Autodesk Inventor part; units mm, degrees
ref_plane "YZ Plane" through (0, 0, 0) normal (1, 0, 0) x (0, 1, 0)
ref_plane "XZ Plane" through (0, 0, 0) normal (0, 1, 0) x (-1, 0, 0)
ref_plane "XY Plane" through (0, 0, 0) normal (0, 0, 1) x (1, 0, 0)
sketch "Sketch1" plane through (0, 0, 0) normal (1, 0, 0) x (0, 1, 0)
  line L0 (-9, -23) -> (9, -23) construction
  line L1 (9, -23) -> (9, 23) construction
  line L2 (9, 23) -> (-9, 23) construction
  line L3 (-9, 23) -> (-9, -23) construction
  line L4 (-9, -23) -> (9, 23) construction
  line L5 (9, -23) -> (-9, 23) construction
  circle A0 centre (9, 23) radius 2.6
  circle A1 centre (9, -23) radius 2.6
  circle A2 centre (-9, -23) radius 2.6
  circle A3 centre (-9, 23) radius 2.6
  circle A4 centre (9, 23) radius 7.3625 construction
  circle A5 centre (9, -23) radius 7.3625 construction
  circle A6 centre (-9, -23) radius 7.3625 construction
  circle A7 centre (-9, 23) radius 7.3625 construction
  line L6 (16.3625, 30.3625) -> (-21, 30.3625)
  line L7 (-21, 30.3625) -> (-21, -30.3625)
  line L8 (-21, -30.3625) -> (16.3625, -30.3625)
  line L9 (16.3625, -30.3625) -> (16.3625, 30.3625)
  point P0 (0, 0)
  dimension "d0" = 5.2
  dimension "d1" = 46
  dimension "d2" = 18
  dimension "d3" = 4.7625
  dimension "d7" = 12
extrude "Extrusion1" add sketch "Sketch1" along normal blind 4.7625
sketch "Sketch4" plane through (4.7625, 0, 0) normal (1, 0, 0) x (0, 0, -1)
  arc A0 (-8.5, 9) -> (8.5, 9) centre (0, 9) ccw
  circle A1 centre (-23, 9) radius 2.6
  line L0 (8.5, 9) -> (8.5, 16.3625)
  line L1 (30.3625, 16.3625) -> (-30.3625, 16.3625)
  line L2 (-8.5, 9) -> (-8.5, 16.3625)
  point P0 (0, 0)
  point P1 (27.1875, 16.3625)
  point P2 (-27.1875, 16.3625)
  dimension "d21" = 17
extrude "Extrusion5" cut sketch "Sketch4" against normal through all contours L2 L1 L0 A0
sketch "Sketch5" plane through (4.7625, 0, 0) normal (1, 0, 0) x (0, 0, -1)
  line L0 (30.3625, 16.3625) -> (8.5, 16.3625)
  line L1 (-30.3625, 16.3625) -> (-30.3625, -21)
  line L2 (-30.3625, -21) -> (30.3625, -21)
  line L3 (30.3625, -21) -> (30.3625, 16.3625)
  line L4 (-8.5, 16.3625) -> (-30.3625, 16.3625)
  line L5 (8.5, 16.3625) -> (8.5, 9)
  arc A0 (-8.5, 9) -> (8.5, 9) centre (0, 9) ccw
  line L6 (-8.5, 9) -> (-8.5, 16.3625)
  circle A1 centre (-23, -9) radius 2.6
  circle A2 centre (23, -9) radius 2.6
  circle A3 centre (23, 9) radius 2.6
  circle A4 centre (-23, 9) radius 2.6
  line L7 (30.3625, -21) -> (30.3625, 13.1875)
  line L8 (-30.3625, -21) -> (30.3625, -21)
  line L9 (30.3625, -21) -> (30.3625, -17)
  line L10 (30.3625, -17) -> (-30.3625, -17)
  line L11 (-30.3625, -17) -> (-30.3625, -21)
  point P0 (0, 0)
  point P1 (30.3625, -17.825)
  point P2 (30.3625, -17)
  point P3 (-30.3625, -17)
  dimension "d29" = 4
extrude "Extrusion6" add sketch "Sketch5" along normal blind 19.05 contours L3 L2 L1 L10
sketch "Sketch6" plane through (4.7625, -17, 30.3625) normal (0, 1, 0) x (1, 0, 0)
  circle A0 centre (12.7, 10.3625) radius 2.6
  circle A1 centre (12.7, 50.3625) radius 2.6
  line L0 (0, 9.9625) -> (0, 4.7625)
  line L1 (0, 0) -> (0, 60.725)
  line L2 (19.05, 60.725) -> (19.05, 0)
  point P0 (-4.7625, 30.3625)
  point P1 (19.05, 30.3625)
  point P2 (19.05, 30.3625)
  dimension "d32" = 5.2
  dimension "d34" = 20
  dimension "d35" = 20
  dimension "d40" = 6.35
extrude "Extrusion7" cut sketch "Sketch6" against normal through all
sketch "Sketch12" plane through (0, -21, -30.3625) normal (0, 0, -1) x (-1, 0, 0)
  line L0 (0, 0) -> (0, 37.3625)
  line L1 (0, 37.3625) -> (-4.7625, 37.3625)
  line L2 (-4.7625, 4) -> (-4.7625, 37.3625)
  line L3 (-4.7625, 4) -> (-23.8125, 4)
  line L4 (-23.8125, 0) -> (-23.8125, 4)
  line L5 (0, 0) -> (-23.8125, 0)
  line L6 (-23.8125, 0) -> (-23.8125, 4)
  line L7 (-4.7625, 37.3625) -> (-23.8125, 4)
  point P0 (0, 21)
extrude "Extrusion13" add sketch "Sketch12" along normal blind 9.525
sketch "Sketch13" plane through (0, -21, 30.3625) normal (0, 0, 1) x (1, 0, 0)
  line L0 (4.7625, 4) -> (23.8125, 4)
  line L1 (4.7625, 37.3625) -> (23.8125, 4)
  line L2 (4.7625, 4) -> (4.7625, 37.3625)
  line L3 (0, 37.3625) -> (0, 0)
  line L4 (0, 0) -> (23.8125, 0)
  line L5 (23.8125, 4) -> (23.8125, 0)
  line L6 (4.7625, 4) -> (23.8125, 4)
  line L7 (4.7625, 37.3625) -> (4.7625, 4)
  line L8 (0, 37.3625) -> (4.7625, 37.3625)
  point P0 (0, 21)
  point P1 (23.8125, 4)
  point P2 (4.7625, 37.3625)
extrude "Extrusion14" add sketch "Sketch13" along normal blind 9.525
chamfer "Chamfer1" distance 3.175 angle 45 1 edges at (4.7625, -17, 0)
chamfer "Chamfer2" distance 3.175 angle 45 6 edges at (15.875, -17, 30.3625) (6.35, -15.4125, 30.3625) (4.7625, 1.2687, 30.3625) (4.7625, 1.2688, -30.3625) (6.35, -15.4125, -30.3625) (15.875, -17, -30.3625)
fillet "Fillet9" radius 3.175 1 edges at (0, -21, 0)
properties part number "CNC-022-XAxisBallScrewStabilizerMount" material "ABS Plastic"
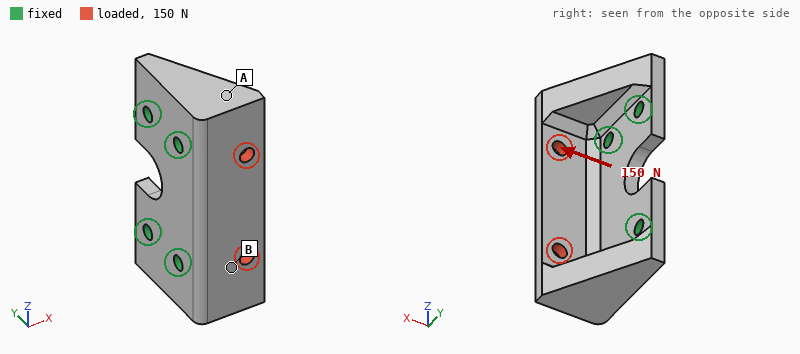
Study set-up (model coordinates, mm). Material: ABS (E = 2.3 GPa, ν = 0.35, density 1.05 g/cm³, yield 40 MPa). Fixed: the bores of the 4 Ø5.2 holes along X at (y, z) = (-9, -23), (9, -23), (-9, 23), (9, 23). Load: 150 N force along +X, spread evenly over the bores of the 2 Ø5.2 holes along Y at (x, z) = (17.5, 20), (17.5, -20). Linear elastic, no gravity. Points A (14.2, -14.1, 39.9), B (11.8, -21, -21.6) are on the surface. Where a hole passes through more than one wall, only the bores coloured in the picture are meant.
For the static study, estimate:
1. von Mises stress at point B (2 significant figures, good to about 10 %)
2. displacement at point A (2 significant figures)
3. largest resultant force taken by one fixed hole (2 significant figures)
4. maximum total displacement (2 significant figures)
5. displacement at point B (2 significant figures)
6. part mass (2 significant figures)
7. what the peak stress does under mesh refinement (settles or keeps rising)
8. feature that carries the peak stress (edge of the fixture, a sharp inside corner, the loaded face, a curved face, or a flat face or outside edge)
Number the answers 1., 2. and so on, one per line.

1. 1.5 MPa
2. 17 µm
3. 96 N
4. 66 µm
5. 40 µm
6. 26 g
7. keeps rising
8. edge of the fixture
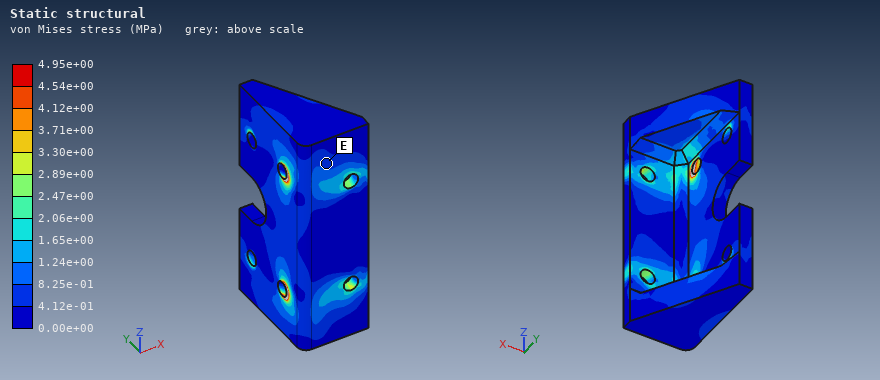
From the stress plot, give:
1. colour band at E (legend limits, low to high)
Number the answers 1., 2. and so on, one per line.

1. 4.12e-01 to 8.25e-01 MPa
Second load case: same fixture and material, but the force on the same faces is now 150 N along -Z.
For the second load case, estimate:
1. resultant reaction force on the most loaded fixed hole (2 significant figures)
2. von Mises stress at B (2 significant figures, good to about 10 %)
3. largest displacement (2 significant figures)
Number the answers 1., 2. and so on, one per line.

1. 90 N
2. 1.1 MPa
3. 49 µm
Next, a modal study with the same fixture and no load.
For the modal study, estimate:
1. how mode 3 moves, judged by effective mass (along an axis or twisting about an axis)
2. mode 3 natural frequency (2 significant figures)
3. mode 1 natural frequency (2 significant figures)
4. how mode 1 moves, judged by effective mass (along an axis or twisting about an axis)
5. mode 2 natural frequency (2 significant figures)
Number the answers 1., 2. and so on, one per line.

1. along X
2. 3500 Hz
3. 2400 Hz
4. along Y
5. 2700 Hz
